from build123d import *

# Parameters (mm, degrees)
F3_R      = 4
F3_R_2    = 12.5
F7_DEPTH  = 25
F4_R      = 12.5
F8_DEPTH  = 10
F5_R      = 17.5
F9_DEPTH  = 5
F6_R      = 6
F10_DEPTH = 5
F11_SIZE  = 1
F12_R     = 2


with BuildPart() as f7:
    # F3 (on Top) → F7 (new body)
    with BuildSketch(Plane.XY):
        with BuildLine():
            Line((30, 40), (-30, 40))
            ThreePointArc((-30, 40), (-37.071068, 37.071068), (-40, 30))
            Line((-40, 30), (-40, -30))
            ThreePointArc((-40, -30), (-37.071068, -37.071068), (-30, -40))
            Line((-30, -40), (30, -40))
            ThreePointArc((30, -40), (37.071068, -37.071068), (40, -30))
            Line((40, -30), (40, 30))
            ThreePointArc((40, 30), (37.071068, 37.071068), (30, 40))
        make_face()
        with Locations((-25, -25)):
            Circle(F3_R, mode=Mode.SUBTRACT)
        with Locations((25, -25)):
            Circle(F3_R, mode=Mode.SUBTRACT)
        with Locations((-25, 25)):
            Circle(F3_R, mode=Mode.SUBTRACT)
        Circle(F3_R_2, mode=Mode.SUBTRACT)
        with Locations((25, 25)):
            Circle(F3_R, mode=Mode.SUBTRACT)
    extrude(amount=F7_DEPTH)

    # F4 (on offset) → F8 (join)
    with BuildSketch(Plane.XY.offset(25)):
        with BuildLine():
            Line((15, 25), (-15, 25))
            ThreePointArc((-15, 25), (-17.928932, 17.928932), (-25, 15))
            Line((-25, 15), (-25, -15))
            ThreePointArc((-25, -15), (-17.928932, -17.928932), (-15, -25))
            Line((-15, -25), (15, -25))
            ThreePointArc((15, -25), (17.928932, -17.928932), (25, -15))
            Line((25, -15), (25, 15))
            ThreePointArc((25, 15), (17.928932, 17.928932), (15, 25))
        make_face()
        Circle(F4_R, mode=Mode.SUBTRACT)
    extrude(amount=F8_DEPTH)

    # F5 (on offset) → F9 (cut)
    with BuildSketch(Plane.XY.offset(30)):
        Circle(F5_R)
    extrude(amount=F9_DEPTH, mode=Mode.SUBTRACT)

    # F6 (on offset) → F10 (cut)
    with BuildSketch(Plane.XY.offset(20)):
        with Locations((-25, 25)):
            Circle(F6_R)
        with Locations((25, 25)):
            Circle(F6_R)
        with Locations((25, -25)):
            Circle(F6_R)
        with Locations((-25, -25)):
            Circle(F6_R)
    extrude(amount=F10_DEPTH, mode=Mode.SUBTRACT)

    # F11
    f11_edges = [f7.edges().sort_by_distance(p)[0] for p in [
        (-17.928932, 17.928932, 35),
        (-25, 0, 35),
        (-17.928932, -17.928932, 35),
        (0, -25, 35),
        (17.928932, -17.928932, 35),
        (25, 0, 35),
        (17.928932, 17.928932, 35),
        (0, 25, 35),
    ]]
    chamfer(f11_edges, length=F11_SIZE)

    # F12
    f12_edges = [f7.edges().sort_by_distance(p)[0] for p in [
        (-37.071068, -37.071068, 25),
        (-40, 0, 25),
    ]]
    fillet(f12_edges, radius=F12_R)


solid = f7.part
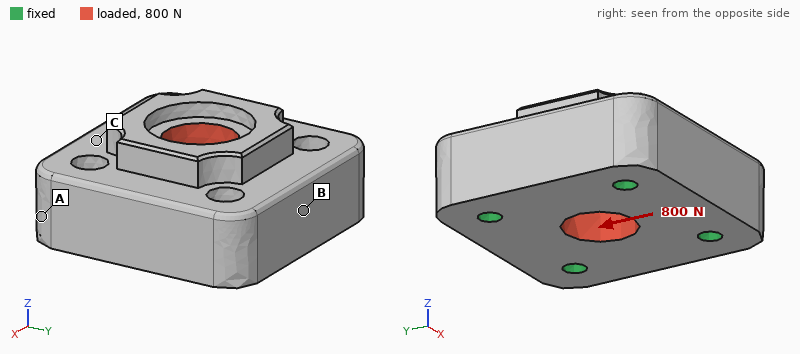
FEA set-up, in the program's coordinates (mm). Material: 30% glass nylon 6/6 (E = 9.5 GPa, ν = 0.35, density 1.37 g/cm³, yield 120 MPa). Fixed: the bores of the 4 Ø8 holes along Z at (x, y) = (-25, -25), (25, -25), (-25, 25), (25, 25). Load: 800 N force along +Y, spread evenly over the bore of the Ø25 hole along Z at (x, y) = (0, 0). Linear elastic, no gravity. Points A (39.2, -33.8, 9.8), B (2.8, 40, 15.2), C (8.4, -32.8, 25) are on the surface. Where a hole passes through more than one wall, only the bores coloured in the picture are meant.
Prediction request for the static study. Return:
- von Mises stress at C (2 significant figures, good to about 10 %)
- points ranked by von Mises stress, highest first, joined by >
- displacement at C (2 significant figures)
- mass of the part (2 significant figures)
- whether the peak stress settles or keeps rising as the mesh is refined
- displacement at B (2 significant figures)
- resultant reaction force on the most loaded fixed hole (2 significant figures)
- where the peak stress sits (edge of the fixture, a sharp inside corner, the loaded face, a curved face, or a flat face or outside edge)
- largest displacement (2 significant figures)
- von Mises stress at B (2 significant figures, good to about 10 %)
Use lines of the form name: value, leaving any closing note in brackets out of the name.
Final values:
von Mises stress at C: 0.17 MPa
points ranked by von Mises stress, highest first, joined by >: B > C > A
displacement at C: 1.2 µm
mass of the part: 210 g
whether the peak stress settles or keeps rising as the mesh is refined: keeps rising
displacement at B: 1.1 µm
resultant reaction force on the most loaded fixed hole: 210 N
where the peak stress sits: edge of the fixture
largest displacement: 1.8 µm
von Mises stress at B: 0.30 MPa
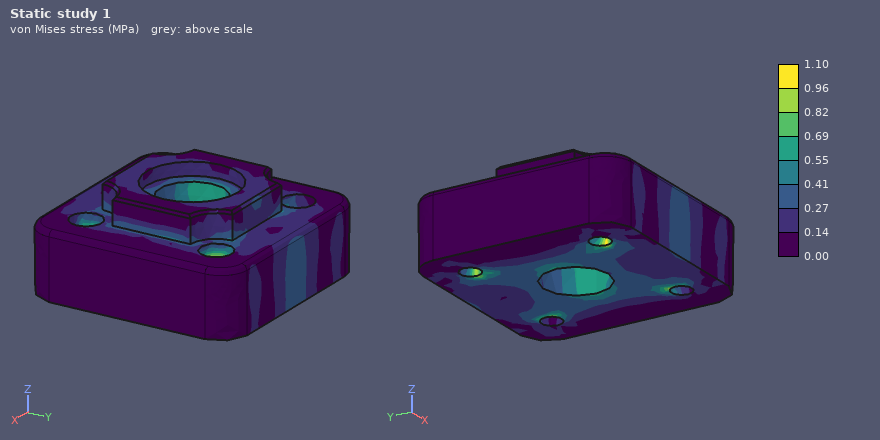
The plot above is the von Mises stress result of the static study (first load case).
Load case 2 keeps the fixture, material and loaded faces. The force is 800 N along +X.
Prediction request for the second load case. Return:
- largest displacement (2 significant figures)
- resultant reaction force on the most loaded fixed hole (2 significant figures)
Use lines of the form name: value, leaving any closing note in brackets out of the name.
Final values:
largest displacement: 1.8 µm
resultant reaction force on the most loaded fixed hole: 210 N
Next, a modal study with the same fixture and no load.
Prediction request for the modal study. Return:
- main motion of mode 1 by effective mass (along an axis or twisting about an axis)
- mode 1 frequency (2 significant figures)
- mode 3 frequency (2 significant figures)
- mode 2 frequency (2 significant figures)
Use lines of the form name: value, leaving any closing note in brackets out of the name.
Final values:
main motion of mode 1 by effective mass: along Z
mode 1 frequency: 11 kHz
mode 3 frequency: 11 kHz
mode 2 frequency: 11 kHz
